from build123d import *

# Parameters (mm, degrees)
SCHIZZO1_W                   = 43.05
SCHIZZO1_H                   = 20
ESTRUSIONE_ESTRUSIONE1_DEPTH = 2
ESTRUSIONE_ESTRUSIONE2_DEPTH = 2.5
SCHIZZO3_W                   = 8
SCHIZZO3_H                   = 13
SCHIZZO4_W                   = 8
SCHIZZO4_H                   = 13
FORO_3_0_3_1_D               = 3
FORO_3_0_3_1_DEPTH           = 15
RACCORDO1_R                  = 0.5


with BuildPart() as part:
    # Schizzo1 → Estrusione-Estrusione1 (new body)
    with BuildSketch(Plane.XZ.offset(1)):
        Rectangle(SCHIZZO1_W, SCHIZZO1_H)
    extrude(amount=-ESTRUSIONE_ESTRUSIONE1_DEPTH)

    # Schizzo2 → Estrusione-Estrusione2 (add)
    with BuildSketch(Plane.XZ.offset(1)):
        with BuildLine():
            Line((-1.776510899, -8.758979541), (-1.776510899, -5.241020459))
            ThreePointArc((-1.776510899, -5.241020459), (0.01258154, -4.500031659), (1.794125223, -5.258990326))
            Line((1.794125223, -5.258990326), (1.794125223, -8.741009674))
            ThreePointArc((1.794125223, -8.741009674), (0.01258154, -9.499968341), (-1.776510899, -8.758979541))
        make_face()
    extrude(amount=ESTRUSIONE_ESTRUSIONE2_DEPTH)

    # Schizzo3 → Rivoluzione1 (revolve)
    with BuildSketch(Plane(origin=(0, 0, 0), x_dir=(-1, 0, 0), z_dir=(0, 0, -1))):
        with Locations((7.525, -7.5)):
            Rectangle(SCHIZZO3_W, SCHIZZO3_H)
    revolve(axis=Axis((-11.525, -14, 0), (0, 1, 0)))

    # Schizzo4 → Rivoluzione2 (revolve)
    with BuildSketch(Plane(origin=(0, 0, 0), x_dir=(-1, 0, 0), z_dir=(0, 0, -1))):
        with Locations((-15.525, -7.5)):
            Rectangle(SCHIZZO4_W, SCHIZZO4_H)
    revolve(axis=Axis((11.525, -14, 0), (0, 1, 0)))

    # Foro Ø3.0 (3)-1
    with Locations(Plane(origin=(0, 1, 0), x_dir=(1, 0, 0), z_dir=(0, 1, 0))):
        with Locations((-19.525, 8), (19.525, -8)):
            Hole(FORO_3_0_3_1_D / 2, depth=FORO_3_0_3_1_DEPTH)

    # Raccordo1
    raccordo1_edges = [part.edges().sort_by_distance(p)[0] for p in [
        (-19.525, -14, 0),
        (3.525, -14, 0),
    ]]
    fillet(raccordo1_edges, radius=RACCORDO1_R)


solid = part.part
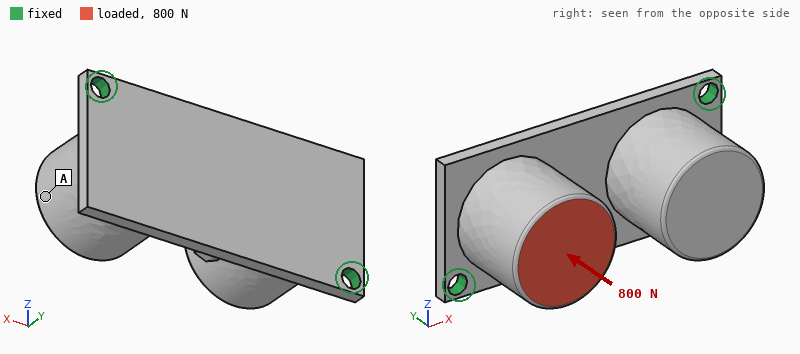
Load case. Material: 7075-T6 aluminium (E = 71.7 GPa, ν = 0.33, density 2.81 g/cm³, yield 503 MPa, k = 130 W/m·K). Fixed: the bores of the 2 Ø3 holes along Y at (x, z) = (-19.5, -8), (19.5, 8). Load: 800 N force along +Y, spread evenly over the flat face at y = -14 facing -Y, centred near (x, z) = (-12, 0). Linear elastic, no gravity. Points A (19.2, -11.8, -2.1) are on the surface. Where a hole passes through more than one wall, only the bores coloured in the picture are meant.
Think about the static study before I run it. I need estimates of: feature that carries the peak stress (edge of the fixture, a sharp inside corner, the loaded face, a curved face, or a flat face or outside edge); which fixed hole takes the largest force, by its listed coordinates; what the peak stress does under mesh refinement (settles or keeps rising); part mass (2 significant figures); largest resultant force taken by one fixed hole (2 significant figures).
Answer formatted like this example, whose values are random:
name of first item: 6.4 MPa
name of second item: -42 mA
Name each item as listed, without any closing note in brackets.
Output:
feature that carries the peak stress: edge of the fixture
which fixed hole takes the largest force, by its listed coordinates: (-19.5, -8)
what the peak stress does under mesh refinement: keeps rising
part mass: 20 g
largest resultant force taken by one fixed hole: 630 N
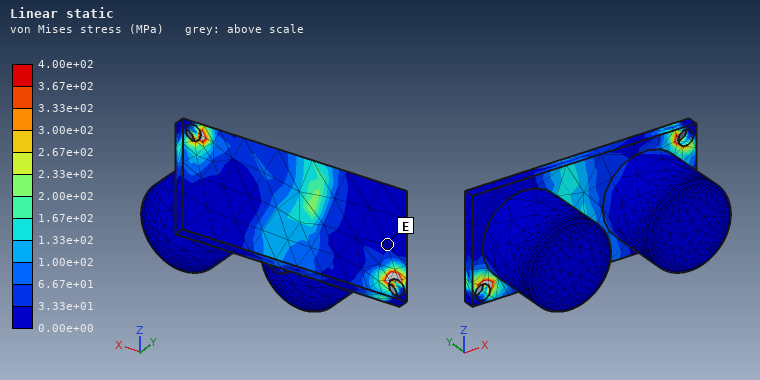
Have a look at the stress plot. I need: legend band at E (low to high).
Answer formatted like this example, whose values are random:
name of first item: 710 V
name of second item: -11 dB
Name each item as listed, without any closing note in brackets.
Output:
legend band at E: 0.00e+00 to 3.33e+01 MPa
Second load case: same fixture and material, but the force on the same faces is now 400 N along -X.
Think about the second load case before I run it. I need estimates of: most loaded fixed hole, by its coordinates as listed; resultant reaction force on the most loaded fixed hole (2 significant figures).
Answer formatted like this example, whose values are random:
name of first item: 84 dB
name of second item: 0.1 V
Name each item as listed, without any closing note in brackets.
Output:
most loaded fixed hole, by its coordinates as listed: (-19.5, -8)
resultant reaction force on the most loaded fixed hole: 270 N
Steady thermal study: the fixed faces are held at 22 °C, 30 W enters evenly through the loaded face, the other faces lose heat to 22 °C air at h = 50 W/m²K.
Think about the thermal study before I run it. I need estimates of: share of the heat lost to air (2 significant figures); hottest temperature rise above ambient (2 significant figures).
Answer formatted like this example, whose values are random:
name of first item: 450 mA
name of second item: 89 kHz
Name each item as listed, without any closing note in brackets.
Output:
share of the heat lost to air: 14 %
hottest temperature rise above ambient: 55 K
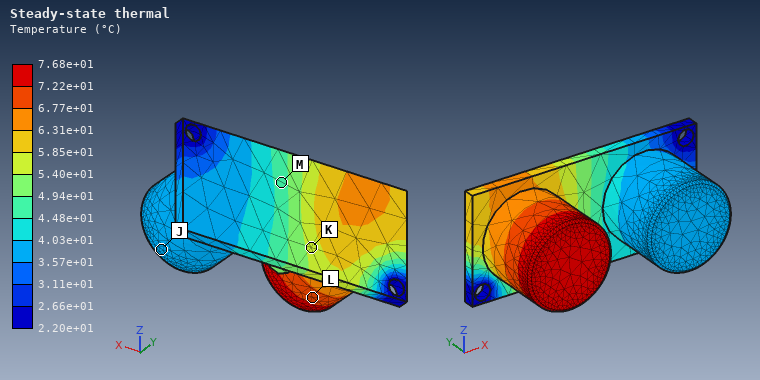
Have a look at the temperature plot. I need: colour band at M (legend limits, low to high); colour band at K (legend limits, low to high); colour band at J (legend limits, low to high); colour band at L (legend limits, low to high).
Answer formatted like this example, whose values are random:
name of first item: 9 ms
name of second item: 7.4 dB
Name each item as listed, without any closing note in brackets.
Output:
colour band at M: 4.48e+01 to 4.94e+01 °C
colour band at K: 5.40e+01 to 5.85e+01 °C
colour band at J: 3.57e+01 to 4.03e+01 °C
colour band at L: 6.77e+01 to 7.22e+01 °C
